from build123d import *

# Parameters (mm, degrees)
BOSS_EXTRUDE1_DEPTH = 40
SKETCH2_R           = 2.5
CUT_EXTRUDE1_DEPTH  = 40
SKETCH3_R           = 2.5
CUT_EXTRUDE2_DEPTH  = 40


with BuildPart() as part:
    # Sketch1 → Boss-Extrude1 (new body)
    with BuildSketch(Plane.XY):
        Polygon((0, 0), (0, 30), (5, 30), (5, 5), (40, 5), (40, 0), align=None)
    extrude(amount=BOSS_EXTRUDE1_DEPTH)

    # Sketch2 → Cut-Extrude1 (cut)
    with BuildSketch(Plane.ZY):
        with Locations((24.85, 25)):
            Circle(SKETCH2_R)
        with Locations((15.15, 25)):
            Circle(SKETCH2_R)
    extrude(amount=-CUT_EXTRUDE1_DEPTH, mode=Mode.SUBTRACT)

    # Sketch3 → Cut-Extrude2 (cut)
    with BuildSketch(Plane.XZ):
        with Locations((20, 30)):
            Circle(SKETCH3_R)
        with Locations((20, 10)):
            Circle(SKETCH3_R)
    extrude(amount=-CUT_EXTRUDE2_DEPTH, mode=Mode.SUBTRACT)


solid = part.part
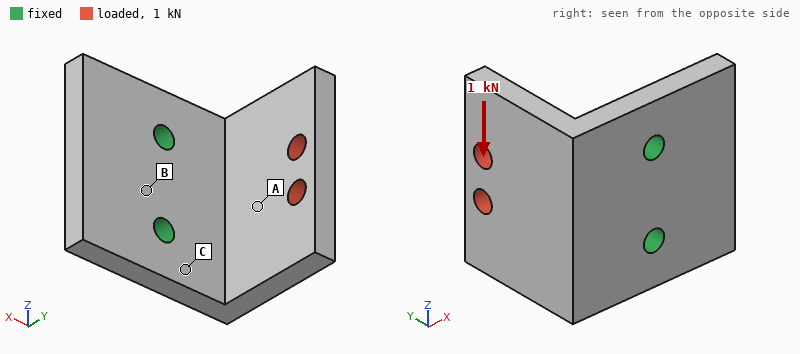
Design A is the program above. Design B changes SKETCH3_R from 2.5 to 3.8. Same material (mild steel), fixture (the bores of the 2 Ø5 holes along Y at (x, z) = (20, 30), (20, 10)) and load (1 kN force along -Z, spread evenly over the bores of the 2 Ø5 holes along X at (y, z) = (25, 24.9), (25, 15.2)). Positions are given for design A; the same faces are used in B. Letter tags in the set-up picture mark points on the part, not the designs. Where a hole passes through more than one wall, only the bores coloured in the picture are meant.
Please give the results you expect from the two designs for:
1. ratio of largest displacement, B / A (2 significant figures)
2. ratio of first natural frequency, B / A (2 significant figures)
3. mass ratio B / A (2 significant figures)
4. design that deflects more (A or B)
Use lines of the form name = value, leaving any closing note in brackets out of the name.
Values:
ratio of largest displacement, B / A = 0.83
ratio of first natural frequency, B / A = 1.1
mass ratio B / A = 0.98
design that deflects more = A
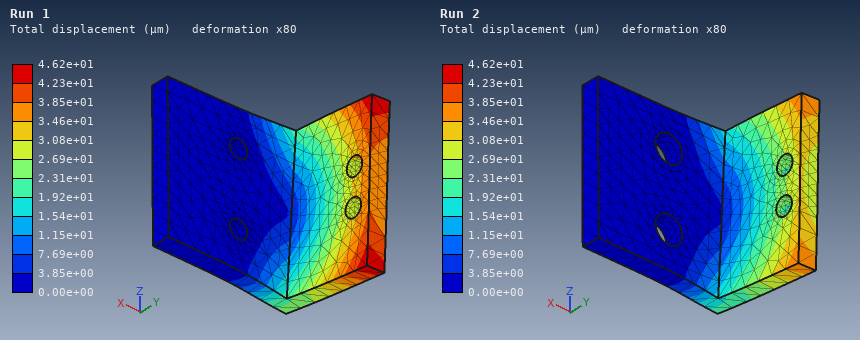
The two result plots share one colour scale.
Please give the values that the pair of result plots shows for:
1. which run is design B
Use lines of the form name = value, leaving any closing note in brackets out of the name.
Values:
which run is design B = Run 2
